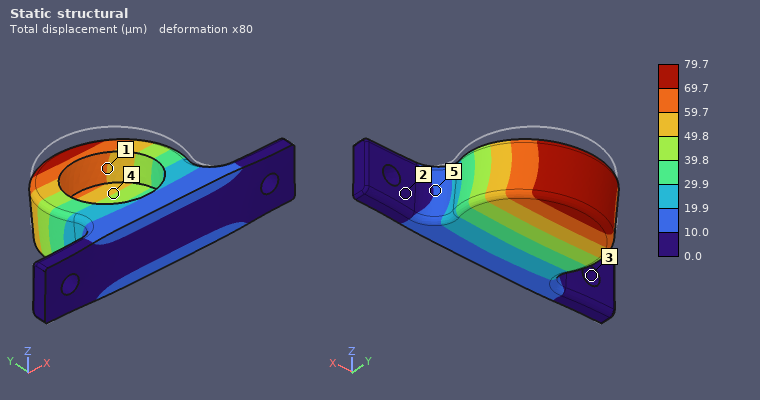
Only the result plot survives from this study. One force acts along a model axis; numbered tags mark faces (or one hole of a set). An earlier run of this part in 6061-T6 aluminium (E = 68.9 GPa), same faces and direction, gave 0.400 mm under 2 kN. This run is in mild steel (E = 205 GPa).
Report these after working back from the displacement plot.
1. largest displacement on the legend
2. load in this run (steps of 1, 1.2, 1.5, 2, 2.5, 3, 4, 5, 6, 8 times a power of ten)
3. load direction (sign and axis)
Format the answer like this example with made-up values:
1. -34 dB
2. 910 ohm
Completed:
1. 79.7 µm
2. 1.2 kN
3. -Z
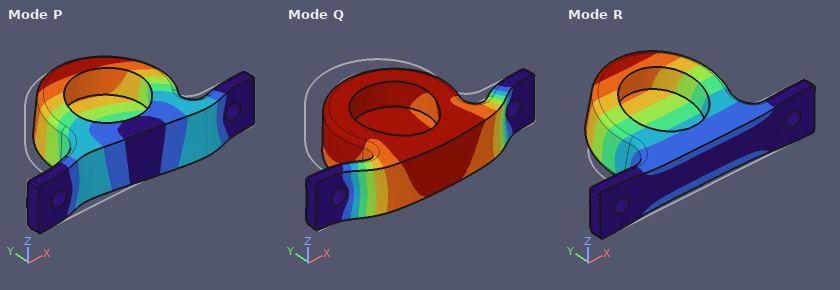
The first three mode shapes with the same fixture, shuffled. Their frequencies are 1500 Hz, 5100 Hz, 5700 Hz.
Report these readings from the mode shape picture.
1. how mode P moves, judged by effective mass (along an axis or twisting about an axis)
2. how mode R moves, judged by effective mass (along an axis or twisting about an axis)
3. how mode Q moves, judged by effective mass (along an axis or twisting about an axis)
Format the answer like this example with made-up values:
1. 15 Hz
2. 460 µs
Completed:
1. along X
2. along Z
3. along Y
